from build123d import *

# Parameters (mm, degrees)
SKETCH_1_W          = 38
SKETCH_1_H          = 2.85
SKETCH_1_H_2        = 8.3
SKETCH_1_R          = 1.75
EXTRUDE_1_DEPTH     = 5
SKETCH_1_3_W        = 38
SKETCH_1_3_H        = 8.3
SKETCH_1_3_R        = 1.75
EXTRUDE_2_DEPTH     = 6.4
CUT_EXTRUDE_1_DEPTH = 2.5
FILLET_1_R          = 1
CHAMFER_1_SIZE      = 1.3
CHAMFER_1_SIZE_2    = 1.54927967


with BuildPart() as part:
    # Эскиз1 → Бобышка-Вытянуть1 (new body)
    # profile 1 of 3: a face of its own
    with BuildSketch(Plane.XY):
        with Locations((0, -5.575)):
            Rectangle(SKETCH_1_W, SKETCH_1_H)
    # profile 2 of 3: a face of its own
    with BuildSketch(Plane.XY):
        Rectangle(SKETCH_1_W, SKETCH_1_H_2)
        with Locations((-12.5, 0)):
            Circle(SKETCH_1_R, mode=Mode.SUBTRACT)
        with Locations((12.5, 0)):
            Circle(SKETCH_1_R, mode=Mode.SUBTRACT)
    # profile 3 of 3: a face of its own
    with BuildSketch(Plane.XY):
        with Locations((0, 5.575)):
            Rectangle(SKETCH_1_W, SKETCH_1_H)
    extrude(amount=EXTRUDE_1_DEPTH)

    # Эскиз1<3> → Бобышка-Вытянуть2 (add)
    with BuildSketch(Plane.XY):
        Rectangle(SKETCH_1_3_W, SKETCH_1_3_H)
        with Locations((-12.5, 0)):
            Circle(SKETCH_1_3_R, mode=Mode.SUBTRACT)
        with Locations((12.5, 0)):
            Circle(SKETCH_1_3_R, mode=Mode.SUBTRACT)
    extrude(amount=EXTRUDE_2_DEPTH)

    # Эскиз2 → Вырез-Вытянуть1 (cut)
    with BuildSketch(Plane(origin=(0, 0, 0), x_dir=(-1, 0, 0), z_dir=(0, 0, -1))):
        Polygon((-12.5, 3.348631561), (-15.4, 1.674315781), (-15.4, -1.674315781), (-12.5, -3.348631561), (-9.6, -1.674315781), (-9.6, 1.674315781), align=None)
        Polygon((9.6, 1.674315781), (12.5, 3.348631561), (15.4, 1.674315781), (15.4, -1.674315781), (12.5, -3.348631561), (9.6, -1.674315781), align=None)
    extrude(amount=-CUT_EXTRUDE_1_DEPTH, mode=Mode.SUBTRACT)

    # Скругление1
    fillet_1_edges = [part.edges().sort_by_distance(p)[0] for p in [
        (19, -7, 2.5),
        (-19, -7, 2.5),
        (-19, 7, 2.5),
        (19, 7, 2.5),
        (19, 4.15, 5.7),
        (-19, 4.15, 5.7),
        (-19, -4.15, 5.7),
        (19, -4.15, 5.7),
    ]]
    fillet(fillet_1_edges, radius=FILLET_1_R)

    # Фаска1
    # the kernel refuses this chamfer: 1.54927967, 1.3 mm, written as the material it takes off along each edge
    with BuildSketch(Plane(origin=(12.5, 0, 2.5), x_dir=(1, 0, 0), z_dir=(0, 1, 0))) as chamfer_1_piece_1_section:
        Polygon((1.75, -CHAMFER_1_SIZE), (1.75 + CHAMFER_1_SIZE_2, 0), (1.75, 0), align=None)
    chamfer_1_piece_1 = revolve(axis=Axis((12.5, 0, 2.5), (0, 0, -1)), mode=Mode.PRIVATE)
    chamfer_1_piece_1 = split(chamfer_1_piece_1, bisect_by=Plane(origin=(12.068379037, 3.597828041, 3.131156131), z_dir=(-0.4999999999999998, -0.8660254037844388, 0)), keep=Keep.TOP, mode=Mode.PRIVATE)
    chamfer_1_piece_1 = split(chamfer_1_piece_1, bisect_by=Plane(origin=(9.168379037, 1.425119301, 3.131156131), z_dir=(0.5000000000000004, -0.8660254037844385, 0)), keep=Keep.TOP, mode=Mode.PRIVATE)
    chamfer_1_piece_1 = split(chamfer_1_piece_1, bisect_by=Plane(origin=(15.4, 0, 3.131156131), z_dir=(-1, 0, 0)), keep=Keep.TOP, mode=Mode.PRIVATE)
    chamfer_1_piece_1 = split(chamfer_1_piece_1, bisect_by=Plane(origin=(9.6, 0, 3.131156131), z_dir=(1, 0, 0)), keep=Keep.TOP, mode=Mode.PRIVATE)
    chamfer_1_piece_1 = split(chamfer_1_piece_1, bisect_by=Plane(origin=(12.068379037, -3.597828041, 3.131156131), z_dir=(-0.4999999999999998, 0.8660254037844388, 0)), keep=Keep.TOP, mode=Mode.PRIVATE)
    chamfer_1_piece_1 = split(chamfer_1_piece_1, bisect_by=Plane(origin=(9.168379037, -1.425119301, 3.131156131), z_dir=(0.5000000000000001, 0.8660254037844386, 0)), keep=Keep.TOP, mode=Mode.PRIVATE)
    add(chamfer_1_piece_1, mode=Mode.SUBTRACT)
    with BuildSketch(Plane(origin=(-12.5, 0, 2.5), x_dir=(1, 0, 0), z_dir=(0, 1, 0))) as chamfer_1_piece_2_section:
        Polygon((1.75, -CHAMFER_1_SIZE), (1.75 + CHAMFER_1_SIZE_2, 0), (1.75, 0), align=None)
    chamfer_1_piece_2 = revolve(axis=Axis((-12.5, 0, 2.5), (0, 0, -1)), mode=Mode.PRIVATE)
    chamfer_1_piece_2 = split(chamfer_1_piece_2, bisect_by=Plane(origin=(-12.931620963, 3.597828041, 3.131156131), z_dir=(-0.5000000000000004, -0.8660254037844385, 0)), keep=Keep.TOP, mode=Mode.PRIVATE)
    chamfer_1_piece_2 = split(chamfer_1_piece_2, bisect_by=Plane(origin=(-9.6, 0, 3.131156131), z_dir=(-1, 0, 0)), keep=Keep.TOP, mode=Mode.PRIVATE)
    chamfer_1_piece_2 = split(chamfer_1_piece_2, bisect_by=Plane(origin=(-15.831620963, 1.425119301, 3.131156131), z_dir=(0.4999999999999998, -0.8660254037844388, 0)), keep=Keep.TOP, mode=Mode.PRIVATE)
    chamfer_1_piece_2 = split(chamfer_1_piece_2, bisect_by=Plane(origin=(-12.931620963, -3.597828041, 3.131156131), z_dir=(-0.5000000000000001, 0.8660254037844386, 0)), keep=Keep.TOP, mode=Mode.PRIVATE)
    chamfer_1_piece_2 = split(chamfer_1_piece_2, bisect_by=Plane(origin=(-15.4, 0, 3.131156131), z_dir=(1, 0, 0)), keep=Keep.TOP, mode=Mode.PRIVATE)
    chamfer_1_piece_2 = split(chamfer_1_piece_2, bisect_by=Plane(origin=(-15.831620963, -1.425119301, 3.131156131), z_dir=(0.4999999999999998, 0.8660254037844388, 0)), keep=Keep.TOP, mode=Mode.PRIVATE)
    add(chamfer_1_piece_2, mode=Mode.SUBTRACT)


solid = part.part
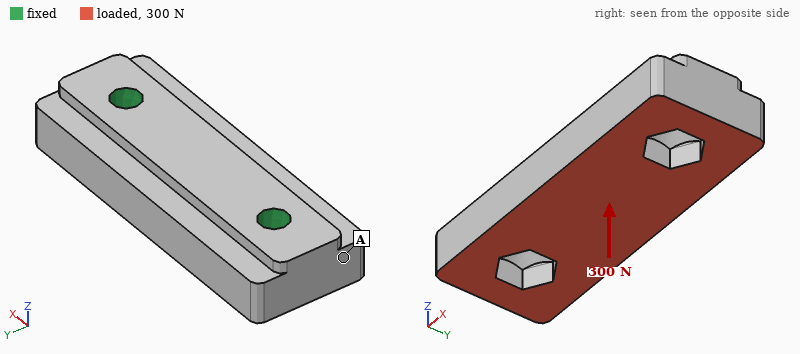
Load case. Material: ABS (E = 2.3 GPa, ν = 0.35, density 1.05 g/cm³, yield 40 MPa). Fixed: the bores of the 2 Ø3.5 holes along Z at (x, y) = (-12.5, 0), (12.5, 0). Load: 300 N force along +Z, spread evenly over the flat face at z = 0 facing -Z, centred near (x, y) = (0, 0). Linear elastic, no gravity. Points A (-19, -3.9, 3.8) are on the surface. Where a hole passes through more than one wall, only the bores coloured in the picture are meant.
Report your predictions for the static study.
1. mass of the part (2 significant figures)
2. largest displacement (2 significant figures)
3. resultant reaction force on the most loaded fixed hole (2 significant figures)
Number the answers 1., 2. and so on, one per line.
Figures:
1. 3.0 g
2. 43 µm
3. 160 N
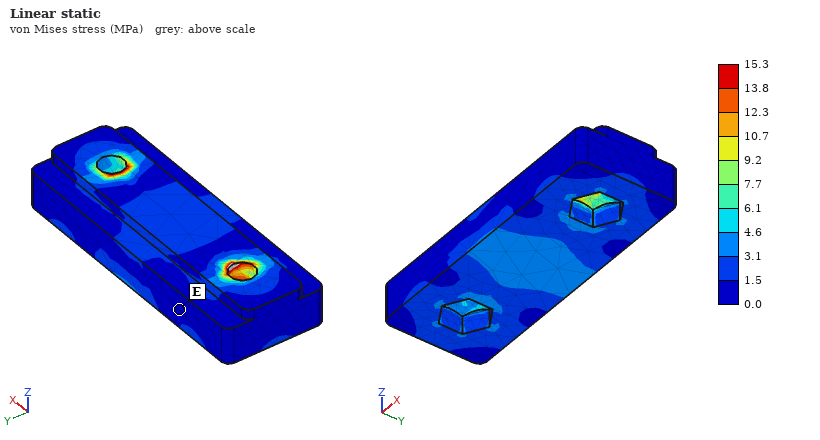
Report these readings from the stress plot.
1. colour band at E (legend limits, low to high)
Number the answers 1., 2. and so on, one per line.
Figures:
1. 0.0 to 1.5 MPa
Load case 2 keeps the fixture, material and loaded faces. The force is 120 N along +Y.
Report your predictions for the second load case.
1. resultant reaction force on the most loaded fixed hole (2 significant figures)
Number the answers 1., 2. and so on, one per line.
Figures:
1. 60 N
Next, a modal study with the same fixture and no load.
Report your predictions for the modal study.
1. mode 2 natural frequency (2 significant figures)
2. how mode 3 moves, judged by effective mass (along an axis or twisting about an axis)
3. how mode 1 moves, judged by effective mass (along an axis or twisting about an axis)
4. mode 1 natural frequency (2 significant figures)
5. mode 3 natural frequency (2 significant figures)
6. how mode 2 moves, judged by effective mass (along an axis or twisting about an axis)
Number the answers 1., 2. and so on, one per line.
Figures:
1. 8400 Hz
2. twisting about Z
3. along Y
4. 6300 Hz
5. 11 kHz
6. along Z
